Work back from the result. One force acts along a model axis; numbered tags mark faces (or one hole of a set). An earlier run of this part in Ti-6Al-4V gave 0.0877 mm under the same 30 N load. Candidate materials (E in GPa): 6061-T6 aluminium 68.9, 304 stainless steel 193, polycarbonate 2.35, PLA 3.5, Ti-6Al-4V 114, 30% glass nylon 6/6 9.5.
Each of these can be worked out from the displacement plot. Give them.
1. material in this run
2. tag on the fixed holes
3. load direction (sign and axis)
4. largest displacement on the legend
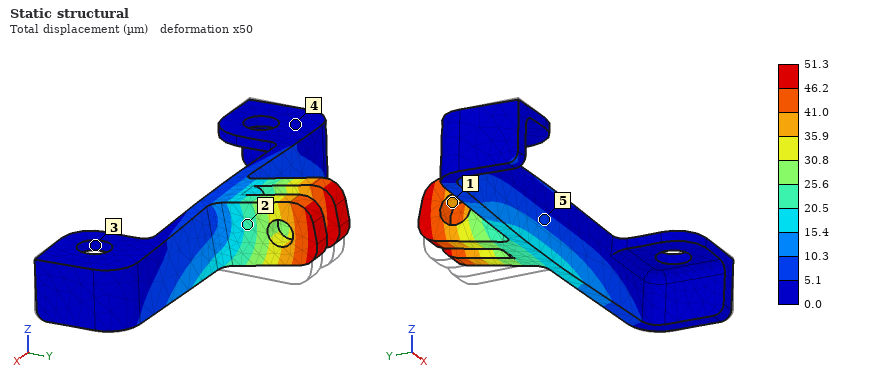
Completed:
304 stainless steel
3
+Z
51.3 µm
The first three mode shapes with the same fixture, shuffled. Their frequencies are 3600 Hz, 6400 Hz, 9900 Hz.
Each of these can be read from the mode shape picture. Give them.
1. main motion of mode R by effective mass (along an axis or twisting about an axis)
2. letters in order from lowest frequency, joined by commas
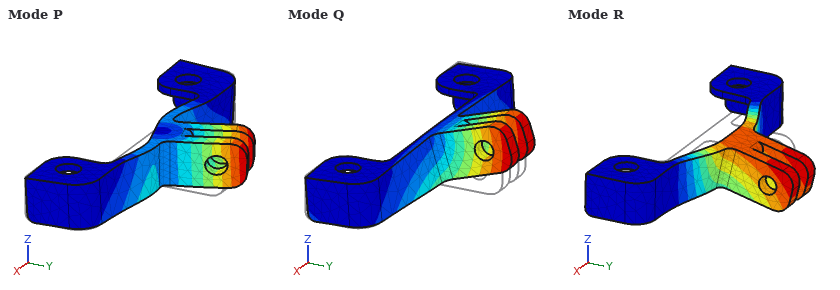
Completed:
along Y
Q, R, P
